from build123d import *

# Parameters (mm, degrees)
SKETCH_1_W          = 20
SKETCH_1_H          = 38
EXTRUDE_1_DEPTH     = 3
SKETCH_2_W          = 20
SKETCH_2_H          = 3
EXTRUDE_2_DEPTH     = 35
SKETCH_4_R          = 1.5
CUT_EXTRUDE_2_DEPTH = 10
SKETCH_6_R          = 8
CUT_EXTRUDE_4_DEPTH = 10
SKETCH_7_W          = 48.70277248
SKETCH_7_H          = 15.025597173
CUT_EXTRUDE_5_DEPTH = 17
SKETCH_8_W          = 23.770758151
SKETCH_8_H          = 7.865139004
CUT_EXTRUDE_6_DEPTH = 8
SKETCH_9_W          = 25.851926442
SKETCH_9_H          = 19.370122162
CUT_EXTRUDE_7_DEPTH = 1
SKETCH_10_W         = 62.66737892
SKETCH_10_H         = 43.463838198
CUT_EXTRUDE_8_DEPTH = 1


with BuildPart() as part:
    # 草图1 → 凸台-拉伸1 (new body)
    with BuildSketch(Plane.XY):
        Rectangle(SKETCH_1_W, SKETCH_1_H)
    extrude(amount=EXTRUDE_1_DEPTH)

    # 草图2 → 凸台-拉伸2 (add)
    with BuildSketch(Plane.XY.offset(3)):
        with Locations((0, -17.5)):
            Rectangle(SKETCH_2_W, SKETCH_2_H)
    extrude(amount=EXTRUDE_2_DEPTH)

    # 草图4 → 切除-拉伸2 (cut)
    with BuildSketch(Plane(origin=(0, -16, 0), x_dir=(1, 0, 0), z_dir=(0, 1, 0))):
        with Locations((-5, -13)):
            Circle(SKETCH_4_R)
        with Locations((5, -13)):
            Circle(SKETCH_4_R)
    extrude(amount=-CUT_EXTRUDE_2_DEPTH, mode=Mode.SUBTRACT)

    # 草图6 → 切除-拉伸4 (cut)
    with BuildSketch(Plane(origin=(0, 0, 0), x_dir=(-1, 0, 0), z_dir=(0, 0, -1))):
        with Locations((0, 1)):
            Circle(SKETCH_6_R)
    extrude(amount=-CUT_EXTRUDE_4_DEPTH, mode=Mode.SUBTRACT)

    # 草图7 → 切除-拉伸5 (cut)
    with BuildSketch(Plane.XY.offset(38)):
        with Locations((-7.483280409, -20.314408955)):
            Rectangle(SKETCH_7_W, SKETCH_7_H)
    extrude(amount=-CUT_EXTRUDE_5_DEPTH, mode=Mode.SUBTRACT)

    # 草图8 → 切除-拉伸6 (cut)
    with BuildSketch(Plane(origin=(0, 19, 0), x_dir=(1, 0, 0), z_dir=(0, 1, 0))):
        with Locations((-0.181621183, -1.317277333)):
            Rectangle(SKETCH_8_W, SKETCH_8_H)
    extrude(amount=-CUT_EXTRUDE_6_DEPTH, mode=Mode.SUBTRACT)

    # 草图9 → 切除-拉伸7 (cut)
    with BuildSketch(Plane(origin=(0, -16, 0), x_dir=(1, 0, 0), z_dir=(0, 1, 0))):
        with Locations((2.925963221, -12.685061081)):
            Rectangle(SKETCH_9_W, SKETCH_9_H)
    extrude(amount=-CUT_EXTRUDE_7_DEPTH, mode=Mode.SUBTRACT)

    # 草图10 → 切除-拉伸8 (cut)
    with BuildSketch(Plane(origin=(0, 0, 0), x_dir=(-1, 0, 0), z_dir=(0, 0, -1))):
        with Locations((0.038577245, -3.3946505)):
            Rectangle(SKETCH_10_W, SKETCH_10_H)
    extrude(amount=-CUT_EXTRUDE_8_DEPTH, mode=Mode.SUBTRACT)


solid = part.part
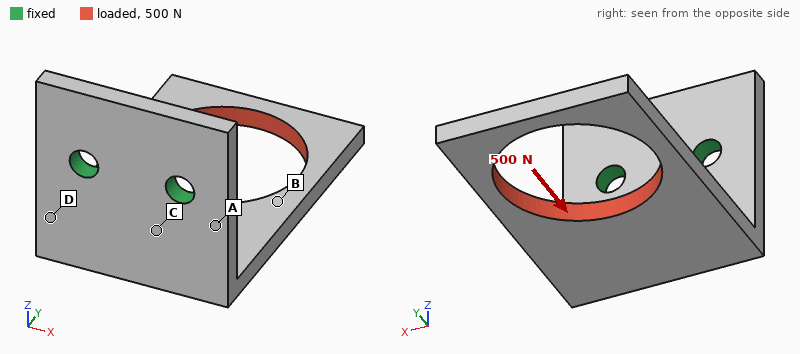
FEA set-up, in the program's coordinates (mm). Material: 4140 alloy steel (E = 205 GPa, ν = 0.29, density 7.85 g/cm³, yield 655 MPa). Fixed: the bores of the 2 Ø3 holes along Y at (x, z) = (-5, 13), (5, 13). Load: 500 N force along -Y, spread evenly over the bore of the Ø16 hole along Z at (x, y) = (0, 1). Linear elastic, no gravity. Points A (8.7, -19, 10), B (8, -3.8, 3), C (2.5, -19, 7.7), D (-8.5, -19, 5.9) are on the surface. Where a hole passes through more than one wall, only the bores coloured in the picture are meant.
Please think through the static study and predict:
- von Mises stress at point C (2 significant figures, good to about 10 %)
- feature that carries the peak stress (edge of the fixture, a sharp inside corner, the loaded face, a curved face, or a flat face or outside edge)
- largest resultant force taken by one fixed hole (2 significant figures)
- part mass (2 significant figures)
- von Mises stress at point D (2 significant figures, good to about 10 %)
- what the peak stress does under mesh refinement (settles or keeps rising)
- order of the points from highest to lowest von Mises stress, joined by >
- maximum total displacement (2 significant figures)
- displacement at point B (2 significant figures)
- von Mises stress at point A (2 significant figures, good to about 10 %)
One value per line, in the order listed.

190 MPa
edge of the fixture
250 N
12 g
140 MPa
keeps rising
A > C > D > B
0.29 mm
0.15 mm
250 MPa
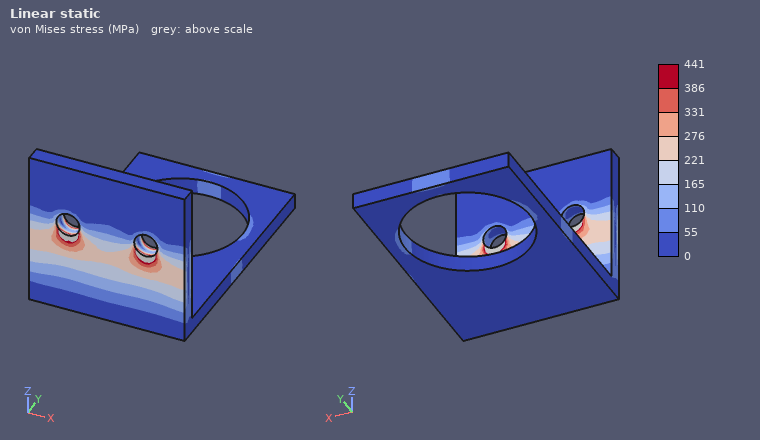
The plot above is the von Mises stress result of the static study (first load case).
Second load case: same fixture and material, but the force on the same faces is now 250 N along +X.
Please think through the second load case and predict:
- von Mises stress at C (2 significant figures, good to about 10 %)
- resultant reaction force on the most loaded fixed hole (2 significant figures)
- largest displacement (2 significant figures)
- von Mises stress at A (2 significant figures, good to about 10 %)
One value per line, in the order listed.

160 MPa
440 N
0.20 mm
180 MPa
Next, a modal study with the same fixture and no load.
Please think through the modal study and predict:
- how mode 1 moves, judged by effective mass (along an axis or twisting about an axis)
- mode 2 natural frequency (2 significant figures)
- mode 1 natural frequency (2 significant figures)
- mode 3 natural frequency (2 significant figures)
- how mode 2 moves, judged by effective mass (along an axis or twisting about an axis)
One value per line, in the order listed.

along Z
3400 Hz
1600 Hz
5100 Hz
along X
